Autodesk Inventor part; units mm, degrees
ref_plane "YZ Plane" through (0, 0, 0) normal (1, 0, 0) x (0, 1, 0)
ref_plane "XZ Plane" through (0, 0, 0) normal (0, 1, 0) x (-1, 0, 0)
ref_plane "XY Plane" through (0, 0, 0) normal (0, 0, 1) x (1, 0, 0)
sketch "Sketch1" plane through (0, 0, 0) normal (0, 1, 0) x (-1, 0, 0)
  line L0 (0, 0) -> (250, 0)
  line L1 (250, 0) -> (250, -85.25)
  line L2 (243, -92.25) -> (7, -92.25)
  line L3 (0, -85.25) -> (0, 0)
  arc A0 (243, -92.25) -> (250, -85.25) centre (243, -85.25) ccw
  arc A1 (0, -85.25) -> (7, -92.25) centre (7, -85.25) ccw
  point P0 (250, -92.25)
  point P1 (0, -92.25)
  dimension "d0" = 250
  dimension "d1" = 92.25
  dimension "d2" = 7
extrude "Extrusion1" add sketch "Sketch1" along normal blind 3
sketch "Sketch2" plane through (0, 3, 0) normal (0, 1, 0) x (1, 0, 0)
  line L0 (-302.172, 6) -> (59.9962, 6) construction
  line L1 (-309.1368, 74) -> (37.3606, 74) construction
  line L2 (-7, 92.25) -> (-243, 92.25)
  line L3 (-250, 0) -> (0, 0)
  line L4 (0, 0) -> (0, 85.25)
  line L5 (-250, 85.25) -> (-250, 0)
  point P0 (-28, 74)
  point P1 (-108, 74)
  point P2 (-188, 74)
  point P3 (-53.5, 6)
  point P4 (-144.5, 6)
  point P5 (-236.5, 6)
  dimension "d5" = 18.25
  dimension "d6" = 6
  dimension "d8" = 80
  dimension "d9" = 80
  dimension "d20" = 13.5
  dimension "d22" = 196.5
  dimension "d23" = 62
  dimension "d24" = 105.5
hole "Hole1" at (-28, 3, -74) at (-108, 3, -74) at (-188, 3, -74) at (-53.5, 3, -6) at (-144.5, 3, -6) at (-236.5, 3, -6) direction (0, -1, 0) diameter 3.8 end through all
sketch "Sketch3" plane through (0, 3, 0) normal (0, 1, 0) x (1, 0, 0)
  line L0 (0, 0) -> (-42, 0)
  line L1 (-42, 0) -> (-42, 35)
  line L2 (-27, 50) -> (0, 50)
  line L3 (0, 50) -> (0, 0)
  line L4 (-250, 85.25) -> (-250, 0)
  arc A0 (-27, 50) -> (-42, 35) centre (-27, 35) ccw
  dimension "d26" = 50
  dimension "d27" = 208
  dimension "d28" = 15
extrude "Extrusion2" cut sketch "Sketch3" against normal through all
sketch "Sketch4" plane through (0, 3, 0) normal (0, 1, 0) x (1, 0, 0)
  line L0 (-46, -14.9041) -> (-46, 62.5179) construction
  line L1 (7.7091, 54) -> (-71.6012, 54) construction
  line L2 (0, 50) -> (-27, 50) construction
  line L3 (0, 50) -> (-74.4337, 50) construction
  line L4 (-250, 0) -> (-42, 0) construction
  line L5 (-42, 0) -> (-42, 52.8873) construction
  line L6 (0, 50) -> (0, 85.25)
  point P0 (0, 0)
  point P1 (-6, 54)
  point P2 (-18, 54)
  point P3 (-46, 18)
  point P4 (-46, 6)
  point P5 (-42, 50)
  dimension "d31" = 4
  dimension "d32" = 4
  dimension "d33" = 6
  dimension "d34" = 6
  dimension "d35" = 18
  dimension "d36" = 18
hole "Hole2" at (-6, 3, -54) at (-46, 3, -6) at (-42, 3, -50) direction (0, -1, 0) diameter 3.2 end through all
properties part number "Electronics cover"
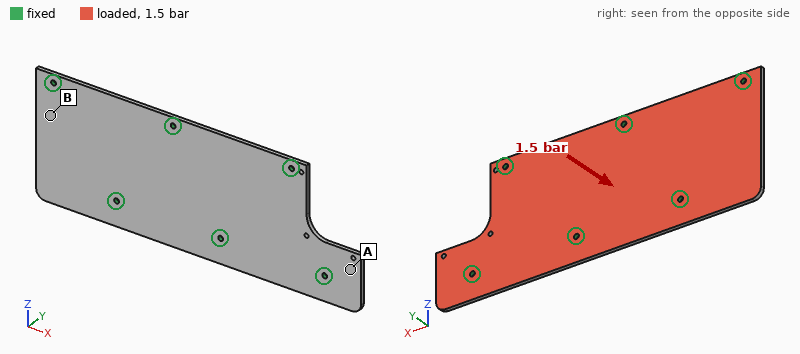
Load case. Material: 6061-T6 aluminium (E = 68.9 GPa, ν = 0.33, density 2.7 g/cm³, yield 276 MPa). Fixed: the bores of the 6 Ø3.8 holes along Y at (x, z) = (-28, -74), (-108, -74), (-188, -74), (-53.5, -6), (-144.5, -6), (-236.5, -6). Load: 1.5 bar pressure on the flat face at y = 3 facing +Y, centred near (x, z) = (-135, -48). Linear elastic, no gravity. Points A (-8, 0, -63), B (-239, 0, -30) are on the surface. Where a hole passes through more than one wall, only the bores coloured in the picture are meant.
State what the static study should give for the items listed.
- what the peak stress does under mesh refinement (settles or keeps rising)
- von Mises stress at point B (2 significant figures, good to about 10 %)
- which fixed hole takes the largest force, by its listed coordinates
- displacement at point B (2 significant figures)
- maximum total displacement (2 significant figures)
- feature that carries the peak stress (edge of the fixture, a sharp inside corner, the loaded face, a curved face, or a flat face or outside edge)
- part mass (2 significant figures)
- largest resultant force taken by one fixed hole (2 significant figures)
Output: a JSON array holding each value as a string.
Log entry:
["keeps rising", "39 MPa", "(-188, -74)", "0.24 mm", "0.96 mm", "edge of the fixture", "170 g", "780 N"]
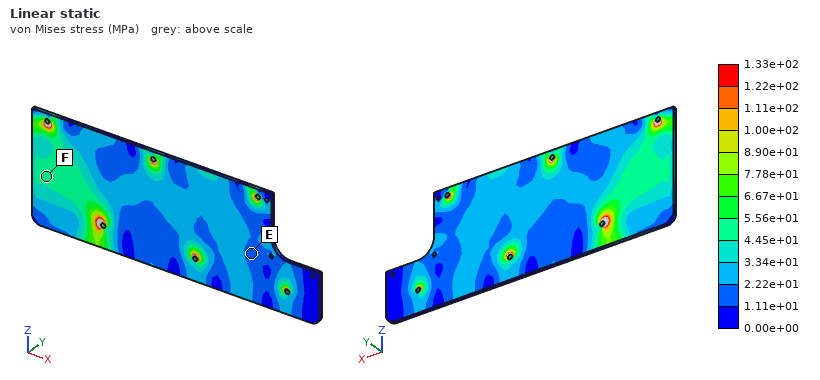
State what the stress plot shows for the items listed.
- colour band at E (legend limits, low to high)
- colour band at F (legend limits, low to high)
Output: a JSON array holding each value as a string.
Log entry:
["1.11e+01 to 2.22e+01 MPa", "4.45e+01 to 5.56e+01 MPa"]
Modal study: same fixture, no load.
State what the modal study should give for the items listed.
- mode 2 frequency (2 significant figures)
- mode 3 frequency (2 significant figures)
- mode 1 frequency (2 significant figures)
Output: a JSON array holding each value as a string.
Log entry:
["1800 Hz", "1800 Hz", "910 Hz"]
